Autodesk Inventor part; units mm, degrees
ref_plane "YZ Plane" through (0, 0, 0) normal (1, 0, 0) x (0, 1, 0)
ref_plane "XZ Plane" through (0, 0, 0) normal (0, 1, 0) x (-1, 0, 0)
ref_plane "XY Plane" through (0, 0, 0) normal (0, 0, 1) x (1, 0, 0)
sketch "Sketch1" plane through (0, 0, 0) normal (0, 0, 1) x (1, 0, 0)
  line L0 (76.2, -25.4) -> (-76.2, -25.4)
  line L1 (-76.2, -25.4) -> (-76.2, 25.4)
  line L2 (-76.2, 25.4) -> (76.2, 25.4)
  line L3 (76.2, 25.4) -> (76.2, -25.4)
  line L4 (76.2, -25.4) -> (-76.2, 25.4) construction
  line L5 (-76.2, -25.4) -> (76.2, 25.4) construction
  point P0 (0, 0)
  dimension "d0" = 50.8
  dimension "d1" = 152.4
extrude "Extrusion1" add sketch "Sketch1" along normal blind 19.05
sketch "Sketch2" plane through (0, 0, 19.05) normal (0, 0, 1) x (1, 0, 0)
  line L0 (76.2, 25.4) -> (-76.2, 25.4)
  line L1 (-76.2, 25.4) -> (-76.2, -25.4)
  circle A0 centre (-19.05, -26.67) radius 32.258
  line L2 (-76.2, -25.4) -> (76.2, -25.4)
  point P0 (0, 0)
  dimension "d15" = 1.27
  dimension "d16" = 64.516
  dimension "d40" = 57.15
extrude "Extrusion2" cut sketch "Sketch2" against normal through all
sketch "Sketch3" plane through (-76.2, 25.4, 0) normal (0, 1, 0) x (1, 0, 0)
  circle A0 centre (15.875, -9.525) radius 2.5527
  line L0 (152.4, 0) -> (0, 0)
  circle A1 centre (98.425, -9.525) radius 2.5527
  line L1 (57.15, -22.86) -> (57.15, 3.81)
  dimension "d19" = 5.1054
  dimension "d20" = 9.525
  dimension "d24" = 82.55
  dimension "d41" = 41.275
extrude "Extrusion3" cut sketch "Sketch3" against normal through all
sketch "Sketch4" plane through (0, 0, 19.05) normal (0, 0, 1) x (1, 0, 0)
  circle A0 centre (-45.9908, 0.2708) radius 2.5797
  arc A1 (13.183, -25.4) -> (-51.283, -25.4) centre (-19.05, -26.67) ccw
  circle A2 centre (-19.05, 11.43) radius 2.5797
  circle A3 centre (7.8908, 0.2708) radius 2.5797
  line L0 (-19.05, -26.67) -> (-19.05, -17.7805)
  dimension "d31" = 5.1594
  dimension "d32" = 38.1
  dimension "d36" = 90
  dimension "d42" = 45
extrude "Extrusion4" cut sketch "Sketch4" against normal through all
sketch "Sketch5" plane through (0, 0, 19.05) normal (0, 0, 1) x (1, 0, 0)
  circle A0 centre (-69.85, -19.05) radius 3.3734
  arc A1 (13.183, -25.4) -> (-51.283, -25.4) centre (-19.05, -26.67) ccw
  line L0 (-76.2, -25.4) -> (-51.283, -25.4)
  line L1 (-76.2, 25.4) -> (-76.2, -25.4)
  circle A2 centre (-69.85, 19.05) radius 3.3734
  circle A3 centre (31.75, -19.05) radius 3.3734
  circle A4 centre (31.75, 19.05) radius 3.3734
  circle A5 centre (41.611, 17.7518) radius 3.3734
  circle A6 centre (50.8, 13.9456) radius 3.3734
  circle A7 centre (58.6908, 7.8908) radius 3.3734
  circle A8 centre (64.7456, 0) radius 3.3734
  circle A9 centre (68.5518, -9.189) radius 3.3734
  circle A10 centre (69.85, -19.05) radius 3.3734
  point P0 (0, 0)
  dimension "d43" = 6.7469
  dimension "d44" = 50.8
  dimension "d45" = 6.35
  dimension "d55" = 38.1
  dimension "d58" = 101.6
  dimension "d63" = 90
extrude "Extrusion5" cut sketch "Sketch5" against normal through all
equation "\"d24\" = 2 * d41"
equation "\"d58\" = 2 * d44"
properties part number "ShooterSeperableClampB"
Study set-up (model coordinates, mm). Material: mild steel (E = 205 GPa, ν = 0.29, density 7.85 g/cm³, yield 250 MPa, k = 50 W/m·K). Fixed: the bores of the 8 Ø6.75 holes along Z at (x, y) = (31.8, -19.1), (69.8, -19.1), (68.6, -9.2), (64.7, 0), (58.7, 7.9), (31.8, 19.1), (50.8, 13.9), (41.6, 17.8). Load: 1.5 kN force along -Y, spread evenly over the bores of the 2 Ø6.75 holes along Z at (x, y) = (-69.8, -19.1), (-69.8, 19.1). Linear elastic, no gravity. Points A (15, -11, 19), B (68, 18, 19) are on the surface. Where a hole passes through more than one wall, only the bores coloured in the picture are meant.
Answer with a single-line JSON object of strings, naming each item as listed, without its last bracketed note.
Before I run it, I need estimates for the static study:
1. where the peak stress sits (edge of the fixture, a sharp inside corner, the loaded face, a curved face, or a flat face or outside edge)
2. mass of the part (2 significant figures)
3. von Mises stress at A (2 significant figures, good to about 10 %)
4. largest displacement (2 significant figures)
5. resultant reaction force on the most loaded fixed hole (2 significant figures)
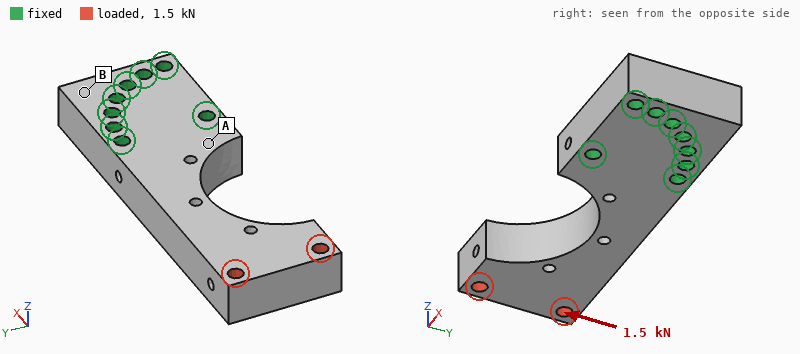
{"where the peak stress sits": "a curved face", "mass of the part": "850 g", "von Mises stress at A": "21 MPa", "largest displacement": "0.12 mm", "resultant reaction force on the most loaded fixed hole": "4.0 kN"}
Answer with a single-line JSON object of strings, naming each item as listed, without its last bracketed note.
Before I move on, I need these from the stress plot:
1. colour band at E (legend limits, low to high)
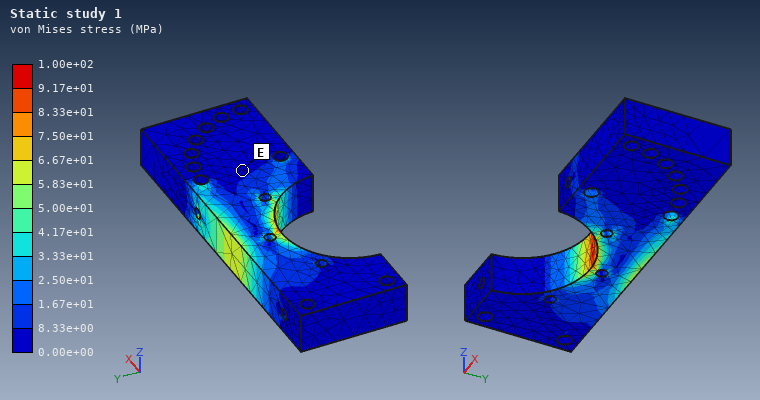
{"colour band at E": "0.00e+00 to 8.33e+00 MPa"}
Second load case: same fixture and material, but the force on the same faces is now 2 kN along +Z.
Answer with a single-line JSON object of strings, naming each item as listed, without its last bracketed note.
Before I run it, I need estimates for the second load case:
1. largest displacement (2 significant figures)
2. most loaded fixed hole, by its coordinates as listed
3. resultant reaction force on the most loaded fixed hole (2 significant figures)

{"largest displacement": "0.30 mm", "most loaded fixed hole, by its coordinates as listed": "(31.8, 19.1)", "resultant reaction force on the most loaded fixed hole": "2.0 kN"}
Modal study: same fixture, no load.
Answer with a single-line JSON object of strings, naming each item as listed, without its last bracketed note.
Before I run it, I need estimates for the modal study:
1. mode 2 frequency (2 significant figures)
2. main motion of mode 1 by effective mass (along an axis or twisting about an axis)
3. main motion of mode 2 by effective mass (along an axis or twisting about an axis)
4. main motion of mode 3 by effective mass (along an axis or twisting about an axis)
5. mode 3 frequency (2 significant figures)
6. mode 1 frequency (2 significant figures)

{"mode 2 frequency": "1500 Hz", "main motion of mode 1 by effective mass": "along Z", "main motion of mode 2 by effective mass": "along Y", "main motion of mode 3 by effective mass": "twisting about X", "mode 3 frequency": "3600 Hz", "mode 1 frequency": "1100 Hz"}
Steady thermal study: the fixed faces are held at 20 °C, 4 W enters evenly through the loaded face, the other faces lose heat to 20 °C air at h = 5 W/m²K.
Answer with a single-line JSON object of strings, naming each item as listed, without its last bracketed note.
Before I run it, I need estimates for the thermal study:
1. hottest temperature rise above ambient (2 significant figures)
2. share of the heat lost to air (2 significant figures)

{"hottest temperature rise above ambient": "16 K", "share of the heat lost to air": "16 %"}
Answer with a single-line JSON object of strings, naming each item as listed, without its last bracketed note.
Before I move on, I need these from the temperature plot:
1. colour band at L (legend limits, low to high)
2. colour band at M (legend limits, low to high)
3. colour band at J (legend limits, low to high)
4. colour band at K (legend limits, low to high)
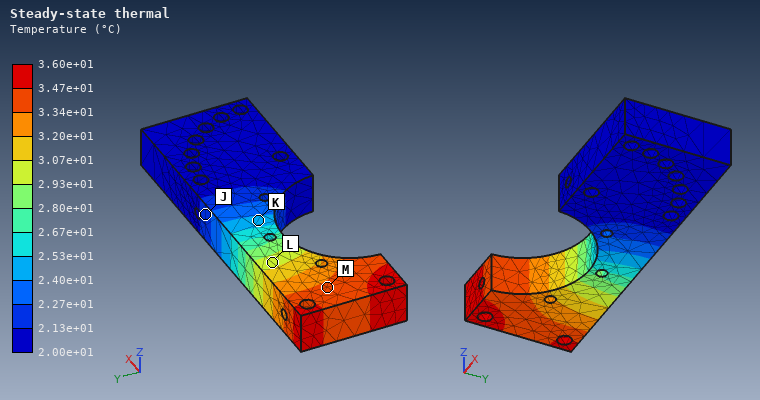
{"colour band at L": "2.93e+01 to 3.07e+01 °C", "colour band at M": "3.34e+01 to 3.47e+01 °C", "colour band at J": "2.13e+01 to 2.27e+01 °C", "colour band at K": "2.40e+01 to 2.53e+01 °C"}
